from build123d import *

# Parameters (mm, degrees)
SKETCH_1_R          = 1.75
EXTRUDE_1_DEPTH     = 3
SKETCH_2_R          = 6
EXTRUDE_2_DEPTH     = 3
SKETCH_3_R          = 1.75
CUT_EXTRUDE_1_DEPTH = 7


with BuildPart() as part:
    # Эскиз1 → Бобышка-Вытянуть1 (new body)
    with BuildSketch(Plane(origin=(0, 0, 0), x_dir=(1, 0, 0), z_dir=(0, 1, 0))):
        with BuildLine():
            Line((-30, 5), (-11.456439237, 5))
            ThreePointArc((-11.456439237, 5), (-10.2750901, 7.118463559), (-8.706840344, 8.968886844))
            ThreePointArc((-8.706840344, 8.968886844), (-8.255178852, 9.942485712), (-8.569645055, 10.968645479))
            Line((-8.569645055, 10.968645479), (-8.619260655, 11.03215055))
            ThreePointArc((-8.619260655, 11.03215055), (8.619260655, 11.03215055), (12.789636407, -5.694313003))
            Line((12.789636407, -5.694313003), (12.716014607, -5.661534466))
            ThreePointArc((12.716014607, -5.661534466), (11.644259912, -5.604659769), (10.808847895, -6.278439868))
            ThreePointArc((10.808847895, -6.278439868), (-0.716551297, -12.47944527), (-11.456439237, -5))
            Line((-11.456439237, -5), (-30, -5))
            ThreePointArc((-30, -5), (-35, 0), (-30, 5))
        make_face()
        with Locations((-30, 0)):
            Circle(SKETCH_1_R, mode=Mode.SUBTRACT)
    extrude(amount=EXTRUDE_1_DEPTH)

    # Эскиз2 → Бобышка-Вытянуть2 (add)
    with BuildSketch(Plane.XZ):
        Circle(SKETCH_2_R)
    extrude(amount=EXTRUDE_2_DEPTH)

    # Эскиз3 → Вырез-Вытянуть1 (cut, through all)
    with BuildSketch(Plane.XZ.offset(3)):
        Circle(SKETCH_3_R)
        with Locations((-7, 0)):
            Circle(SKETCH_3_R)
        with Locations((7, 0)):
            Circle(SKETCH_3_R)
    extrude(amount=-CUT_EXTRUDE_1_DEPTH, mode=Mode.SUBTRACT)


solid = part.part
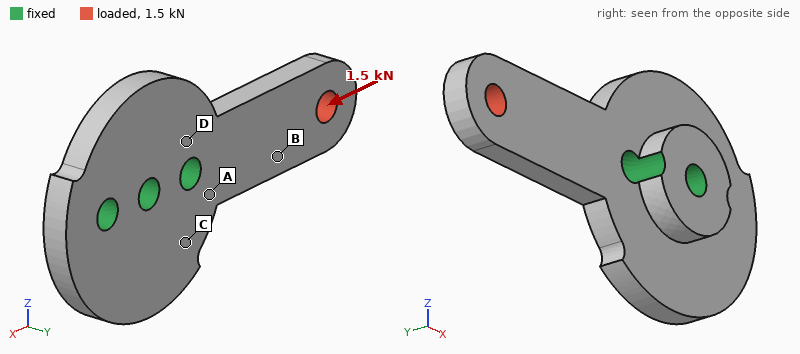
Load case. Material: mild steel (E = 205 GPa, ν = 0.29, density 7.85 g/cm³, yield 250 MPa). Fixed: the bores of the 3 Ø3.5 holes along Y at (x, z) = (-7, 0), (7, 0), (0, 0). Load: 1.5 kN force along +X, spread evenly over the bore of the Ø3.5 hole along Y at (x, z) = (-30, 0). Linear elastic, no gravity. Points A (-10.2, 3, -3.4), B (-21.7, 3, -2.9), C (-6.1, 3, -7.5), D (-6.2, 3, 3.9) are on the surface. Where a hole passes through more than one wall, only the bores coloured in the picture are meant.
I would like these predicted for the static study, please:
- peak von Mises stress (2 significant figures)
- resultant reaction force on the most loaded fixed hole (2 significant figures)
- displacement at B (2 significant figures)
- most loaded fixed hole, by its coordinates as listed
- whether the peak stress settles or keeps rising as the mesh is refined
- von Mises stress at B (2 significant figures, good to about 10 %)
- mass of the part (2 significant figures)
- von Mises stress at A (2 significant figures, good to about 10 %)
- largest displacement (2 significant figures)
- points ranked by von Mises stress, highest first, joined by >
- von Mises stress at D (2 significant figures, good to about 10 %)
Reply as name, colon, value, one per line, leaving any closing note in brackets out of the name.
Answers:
peak von Mises stress: 140 MPa
resultant reaction force on the most loaded fixed hole: 1.2 kN
displacement at B: 3.5 µm
most loaded fixed hole, by its coordinates as listed: (-7, 0)
whether the peak stress settles or keeps rising as the mesh is refined: settles
von Mises stress at B: 50 MPa
mass of the part: 19 g
von Mises stress at A: 35 MPa
largest displacement: 7.0 µm
points ranked by von Mises stress, highest first, joined by >: B > A > D > C
von Mises stress at D: 20 MPa
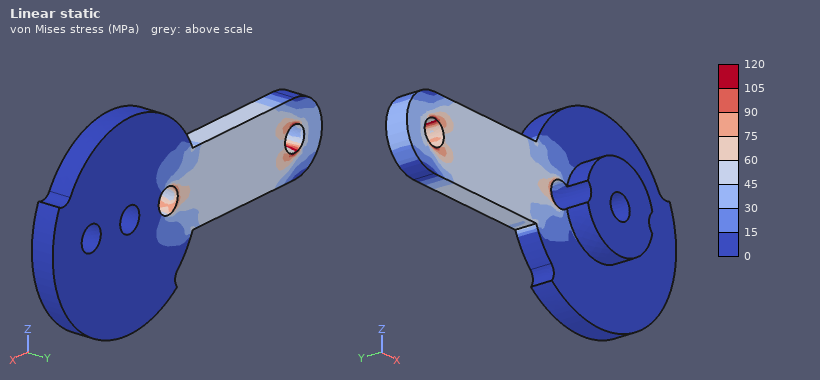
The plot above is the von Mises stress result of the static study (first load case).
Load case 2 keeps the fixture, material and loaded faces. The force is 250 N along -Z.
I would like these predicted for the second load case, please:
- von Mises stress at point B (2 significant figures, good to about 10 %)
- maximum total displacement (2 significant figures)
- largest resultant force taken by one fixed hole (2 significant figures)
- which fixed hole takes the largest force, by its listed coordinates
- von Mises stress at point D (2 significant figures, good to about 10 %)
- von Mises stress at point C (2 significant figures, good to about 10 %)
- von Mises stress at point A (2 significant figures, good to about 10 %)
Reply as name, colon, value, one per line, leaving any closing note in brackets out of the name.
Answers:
von Mises stress at point B: 28 MPa
maximum total displacement: 27 µm
largest resultant force taken by one fixed hole: 500 N
which fixed hole takes the largest force, by its listed coordinates: (-7, 0)
von Mises stress at point D: 32 MPa
von Mises stress at point C: 16 MPa
von Mises stress at point A: 43 MPa
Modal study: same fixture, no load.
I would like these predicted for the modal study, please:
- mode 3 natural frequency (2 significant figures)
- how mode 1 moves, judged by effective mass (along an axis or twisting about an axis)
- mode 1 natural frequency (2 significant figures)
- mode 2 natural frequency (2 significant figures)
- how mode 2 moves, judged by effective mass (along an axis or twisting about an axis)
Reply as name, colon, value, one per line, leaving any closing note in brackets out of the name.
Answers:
mode 3 natural frequency: 17 kHz
how mode 1 moves, judged by effective mass: along Y
mode 1 natural frequency: 3900 Hz
mode 2 natural frequency: 11 kHz
how mode 2 moves, judged by effective mass: along Z
